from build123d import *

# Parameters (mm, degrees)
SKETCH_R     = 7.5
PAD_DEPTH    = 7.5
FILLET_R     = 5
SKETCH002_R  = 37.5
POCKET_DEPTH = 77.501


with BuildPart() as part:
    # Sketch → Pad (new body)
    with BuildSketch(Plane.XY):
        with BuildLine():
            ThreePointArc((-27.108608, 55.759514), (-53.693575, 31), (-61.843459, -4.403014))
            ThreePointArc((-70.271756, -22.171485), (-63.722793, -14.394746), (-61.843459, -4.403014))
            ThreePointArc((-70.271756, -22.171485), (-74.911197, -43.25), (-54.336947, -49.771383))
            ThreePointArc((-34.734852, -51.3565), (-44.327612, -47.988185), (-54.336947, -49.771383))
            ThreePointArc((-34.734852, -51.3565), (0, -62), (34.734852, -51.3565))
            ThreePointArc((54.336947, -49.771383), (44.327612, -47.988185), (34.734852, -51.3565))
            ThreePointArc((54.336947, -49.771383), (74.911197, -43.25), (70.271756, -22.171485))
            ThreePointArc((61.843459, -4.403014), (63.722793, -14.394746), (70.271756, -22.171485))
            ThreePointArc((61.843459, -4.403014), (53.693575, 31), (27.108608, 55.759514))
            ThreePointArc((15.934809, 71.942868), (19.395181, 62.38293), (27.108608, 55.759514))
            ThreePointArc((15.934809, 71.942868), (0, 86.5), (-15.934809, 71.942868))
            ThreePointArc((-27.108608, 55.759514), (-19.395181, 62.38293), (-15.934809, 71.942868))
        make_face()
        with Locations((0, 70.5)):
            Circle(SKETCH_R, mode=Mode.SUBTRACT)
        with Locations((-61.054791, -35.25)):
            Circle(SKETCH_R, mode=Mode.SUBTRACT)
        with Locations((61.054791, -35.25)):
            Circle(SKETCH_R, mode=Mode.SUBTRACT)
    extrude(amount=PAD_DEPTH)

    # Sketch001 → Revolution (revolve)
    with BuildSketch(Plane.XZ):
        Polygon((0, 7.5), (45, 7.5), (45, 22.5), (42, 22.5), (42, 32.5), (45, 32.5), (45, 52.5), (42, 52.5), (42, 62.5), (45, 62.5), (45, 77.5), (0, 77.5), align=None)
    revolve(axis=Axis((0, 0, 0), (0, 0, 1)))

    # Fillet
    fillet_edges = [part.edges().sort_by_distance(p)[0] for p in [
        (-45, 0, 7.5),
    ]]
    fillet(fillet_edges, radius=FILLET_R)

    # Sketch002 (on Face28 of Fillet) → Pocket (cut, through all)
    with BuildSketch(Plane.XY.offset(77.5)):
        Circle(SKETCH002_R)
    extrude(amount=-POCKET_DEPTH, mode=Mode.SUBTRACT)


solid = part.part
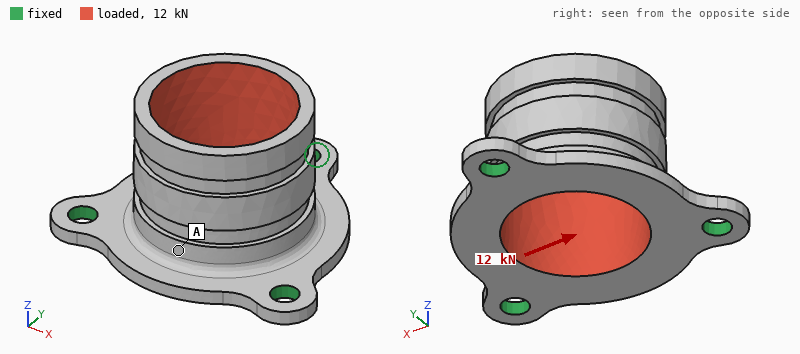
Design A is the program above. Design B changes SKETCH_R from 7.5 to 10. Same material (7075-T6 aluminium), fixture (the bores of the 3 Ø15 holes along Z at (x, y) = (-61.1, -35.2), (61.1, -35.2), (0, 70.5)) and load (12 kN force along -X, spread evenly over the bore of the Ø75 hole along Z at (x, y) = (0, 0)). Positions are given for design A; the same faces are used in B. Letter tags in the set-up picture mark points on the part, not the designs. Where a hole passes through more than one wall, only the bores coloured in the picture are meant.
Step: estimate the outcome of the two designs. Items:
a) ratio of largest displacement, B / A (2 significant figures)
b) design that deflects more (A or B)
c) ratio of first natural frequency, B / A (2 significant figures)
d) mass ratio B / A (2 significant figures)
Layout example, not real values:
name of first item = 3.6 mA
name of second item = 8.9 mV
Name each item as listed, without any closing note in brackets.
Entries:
ratio of largest displacement, B / A = 0.84
design that deflects more = A
ratio of first natural frequency, B / A = 1.1
mass ratio B / A = 0.98
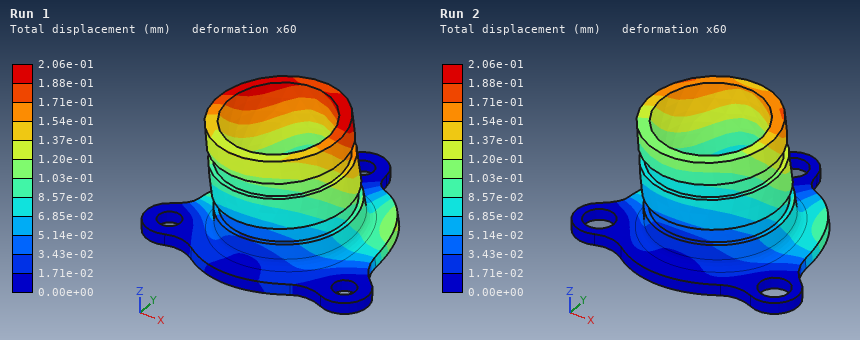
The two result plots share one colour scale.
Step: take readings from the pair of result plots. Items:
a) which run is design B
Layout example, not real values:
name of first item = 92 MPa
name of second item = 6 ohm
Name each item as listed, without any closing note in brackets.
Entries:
which run is design B = Run 2
